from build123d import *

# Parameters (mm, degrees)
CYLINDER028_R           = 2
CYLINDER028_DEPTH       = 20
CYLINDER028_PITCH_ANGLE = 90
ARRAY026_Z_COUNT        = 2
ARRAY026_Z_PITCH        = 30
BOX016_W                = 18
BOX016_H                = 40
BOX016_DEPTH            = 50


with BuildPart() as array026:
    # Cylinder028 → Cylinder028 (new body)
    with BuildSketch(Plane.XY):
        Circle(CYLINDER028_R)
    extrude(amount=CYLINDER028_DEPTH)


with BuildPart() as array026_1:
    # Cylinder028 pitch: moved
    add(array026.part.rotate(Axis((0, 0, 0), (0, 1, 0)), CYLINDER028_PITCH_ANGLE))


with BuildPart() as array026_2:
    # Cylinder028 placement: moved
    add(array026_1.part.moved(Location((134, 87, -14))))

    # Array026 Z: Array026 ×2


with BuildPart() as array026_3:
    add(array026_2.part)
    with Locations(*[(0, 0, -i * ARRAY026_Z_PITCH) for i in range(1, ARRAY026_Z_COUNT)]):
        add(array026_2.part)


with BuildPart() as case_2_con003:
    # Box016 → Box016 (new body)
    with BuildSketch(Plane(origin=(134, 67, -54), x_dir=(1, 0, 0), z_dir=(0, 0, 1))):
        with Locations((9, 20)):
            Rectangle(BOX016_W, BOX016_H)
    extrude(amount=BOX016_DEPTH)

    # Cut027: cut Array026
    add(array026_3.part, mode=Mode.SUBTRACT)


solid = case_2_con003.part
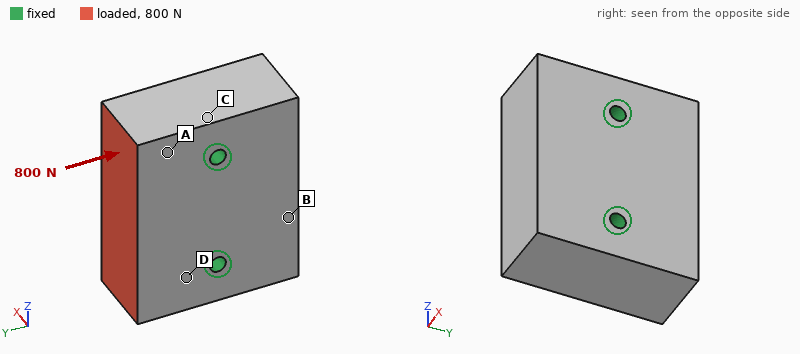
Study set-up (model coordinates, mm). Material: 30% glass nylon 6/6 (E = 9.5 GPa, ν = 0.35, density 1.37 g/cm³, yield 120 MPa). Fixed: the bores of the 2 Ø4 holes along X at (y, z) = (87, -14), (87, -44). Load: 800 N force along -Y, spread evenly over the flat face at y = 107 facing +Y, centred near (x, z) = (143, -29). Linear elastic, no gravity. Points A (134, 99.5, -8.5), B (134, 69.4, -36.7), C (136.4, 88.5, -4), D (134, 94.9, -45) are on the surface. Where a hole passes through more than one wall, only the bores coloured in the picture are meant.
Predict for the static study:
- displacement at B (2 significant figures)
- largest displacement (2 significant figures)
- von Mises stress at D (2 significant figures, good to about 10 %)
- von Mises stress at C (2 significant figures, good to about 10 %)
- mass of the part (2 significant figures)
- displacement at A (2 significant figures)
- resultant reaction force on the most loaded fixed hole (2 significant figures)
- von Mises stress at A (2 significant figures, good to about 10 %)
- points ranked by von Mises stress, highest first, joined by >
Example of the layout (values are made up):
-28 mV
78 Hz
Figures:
0.78 µm
2.6 µm
1.2 MPa
0.51 MPa
49 g
1.8 µm
400 N
0.90 MPa
D > A > C > B
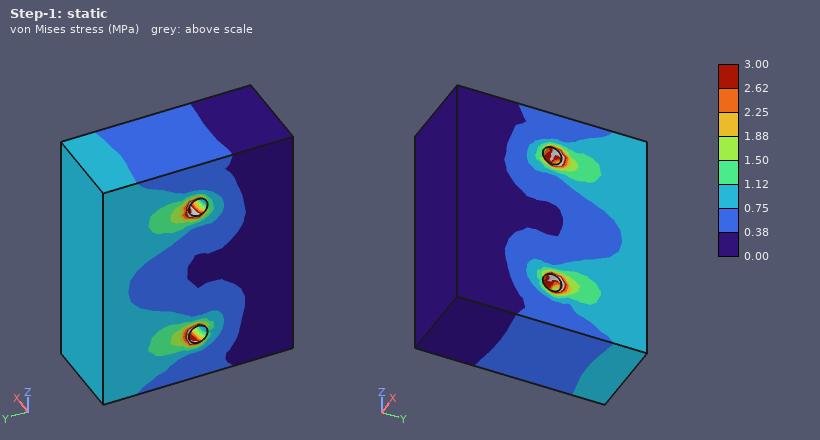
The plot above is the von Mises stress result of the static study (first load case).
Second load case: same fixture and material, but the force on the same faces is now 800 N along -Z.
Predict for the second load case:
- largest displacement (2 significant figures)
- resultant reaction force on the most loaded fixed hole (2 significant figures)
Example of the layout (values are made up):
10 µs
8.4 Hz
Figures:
12 µm
630 N
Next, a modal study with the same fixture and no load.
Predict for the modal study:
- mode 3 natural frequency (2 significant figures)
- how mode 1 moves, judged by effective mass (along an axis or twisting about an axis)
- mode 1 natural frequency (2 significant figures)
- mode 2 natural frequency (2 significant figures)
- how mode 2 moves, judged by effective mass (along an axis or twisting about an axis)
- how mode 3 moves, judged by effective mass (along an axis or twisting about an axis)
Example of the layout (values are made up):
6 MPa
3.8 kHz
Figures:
13 kHz
twisting about Z
9100 Hz
12 kHz
along X
twisting about X
